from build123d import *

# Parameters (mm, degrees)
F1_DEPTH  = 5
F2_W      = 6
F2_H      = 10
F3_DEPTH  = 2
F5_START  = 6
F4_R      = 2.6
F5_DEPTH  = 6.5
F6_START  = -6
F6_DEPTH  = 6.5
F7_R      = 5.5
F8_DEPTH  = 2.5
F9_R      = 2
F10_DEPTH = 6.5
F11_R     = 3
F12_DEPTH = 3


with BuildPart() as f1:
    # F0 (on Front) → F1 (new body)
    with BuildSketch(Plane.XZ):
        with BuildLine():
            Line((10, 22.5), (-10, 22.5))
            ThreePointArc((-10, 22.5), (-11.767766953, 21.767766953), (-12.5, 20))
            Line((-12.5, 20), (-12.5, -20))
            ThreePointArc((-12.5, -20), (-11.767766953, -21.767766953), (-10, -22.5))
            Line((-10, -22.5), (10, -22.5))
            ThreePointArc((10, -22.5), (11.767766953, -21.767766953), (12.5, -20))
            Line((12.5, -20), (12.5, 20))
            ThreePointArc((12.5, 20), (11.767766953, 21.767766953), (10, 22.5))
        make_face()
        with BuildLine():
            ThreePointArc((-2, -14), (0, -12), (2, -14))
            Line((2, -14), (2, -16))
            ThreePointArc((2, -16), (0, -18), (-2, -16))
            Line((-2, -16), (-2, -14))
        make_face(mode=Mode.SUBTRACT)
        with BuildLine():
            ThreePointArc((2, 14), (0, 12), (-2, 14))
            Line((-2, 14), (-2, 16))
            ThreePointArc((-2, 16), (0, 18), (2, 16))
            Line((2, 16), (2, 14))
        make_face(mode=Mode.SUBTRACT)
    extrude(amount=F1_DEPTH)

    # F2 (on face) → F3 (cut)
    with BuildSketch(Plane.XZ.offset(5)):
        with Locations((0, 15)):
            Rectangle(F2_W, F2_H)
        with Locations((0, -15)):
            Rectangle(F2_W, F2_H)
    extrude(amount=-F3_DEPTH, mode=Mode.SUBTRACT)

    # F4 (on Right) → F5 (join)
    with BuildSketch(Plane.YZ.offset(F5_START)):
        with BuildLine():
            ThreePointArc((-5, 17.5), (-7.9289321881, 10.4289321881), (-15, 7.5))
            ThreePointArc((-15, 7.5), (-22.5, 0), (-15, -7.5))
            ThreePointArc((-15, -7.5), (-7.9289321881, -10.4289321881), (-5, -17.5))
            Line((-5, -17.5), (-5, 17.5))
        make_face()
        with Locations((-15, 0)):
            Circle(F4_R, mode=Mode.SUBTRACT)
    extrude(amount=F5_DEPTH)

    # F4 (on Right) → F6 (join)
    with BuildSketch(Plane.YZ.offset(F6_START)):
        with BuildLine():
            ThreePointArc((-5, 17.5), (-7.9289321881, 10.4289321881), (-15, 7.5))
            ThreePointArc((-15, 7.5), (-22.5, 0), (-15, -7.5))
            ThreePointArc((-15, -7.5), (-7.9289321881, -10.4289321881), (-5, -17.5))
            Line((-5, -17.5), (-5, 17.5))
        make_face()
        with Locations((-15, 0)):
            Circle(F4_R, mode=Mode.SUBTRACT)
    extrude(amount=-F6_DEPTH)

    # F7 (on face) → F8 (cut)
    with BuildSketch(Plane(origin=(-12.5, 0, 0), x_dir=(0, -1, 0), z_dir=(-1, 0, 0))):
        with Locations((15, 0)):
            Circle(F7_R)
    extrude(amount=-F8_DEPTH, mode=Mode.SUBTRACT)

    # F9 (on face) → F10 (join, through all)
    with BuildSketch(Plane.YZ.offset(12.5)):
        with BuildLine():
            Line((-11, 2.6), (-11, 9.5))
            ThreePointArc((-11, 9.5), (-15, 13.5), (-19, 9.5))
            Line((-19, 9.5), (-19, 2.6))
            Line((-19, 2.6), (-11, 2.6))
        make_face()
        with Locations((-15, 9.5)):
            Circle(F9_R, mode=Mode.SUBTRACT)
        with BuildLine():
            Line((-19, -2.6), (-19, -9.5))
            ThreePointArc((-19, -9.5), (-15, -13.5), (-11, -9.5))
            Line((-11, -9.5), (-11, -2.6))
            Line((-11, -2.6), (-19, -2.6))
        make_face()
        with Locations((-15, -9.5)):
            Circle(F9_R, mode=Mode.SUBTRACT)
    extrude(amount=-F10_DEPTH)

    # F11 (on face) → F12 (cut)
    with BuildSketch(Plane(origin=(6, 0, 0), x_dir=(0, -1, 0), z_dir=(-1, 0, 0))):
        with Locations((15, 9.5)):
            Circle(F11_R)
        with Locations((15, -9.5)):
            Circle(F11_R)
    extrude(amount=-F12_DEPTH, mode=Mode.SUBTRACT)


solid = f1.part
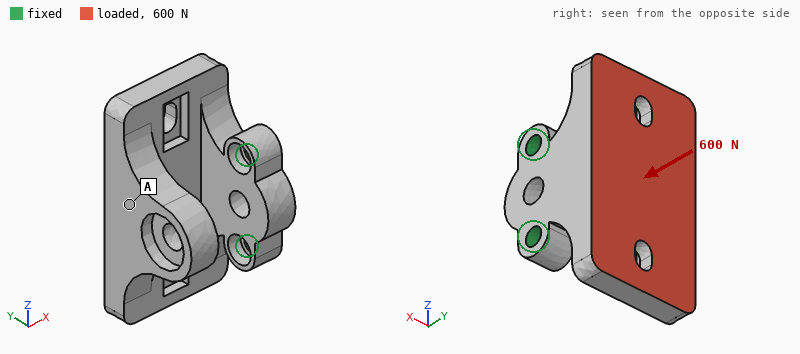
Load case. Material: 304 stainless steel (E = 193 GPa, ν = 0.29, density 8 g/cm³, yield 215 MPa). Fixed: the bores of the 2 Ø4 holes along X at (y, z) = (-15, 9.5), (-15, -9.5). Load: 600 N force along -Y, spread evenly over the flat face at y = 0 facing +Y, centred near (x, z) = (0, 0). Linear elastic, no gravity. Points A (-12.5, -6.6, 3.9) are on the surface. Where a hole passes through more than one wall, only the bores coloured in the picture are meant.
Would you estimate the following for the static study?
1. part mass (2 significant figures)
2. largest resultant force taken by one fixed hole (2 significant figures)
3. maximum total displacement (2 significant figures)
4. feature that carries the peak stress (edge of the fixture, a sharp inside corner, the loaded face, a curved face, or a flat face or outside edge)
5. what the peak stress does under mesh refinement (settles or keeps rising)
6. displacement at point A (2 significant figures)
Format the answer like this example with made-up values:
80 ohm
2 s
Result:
70 g
300 N
50 µm
edge of the fixture
keeps rising
43 µm
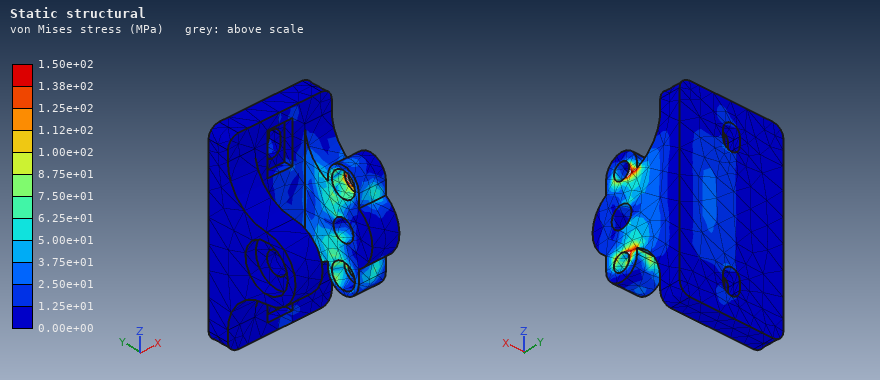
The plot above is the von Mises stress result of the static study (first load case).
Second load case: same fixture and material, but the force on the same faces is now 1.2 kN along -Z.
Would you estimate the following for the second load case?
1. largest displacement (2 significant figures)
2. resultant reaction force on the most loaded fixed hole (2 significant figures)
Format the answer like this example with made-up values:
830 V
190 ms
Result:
28 µm
1.4 kN
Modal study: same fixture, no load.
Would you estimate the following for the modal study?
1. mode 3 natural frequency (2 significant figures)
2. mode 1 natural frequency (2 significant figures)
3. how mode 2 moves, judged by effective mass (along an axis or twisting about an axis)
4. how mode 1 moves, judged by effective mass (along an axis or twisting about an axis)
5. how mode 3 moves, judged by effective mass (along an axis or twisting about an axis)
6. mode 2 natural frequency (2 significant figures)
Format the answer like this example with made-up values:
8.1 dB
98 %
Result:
6400 Hz
2400 Hz
along Z
along Y
along X
3900 Hz
